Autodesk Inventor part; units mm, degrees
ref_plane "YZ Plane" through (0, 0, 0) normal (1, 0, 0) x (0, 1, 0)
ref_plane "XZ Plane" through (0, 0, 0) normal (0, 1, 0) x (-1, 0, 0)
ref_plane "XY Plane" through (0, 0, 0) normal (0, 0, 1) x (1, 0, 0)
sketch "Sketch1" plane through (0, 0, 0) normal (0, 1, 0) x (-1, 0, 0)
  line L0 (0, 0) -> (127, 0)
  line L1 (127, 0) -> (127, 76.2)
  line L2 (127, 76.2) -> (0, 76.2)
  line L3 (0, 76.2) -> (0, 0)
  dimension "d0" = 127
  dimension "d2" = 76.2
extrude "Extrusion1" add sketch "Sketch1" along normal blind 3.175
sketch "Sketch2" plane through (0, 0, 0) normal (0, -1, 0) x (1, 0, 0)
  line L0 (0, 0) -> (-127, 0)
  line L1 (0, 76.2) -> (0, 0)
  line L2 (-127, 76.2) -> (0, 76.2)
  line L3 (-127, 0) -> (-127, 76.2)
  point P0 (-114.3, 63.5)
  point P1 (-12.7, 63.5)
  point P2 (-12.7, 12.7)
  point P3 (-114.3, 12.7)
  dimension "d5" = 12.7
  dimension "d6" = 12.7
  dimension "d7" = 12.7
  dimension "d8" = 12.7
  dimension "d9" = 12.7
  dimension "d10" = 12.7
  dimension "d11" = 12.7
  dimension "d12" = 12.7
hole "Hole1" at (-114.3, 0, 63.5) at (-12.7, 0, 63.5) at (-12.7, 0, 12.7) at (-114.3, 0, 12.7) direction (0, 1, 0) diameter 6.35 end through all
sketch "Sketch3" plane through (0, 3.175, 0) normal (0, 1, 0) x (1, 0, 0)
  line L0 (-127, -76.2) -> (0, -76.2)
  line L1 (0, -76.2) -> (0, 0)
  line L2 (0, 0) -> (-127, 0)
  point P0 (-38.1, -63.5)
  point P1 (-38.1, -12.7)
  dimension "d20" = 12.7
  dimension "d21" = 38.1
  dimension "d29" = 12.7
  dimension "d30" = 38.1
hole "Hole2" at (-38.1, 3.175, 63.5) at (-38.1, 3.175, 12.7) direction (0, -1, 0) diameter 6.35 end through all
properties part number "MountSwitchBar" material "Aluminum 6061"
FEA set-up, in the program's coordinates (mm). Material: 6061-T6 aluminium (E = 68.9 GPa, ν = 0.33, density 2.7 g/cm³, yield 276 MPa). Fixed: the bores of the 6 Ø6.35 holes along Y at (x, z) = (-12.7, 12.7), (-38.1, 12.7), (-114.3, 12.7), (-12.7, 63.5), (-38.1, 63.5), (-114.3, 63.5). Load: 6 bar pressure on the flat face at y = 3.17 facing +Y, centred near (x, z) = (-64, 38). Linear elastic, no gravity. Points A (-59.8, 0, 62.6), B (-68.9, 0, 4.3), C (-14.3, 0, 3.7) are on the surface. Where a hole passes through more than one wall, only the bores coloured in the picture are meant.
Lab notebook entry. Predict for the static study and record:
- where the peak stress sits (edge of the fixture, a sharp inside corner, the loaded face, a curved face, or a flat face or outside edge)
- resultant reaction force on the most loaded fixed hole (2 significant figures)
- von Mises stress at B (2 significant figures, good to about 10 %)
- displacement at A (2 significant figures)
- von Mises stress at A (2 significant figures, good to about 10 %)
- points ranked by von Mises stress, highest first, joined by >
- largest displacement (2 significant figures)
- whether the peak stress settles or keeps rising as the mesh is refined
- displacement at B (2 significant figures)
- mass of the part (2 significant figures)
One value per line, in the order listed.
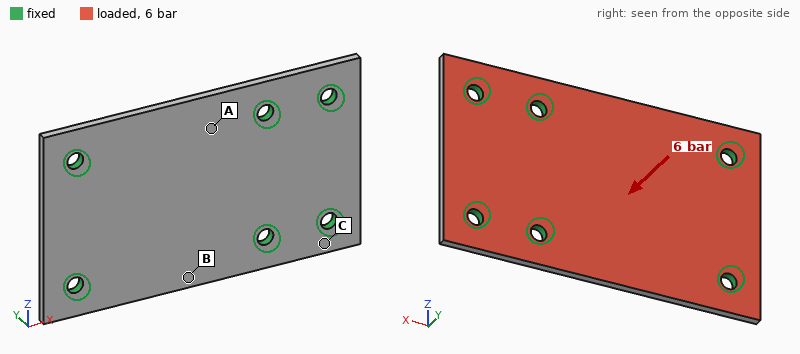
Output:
edge of the fixture
1.2 kN
78 MPa
0.19 mm
43 MPa
B > A > C
0.32 mm
keeps rising
0.26 mm
81 g
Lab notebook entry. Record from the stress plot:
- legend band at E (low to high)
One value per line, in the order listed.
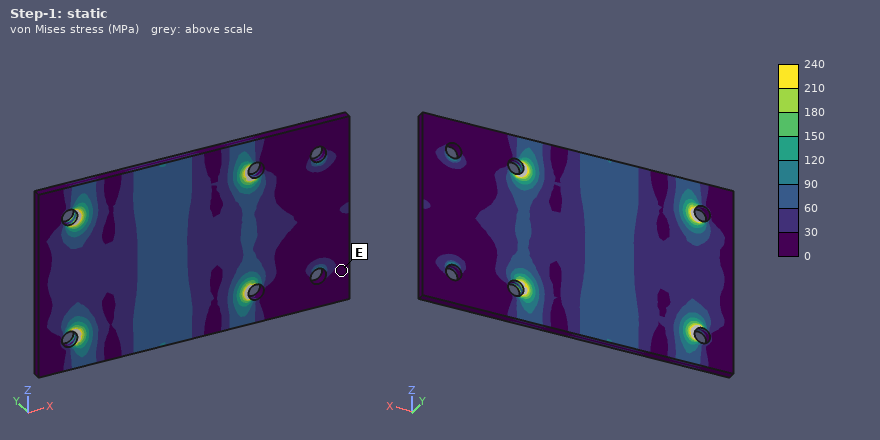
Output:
0 to 30 MPa
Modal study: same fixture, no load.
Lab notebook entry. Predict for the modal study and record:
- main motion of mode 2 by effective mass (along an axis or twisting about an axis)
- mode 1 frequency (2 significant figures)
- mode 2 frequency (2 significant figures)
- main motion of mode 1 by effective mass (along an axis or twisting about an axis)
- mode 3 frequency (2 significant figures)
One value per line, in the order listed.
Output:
twisting about X
2800 Hz
3500 Hz
along Y
4900 Hz
